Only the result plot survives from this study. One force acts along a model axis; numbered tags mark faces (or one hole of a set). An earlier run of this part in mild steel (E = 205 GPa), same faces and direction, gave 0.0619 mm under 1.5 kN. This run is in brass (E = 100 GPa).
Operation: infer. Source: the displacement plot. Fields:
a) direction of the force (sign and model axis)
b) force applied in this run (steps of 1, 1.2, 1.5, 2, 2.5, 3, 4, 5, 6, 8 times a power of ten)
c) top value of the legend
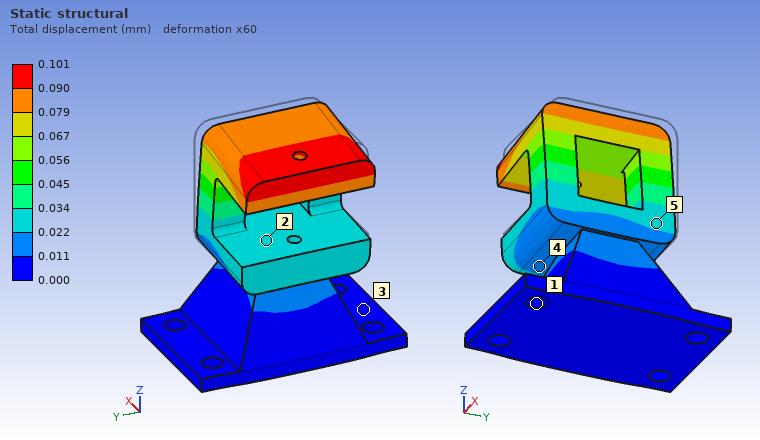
-X
1.2 kN
0.101 mm
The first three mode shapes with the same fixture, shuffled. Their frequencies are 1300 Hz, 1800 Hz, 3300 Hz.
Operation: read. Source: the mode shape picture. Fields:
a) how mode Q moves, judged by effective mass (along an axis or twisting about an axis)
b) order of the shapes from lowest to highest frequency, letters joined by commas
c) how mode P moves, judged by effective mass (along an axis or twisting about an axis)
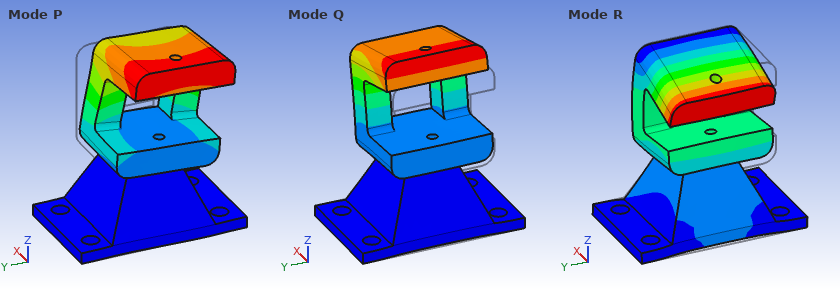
along X
Q, P, R
along Y
